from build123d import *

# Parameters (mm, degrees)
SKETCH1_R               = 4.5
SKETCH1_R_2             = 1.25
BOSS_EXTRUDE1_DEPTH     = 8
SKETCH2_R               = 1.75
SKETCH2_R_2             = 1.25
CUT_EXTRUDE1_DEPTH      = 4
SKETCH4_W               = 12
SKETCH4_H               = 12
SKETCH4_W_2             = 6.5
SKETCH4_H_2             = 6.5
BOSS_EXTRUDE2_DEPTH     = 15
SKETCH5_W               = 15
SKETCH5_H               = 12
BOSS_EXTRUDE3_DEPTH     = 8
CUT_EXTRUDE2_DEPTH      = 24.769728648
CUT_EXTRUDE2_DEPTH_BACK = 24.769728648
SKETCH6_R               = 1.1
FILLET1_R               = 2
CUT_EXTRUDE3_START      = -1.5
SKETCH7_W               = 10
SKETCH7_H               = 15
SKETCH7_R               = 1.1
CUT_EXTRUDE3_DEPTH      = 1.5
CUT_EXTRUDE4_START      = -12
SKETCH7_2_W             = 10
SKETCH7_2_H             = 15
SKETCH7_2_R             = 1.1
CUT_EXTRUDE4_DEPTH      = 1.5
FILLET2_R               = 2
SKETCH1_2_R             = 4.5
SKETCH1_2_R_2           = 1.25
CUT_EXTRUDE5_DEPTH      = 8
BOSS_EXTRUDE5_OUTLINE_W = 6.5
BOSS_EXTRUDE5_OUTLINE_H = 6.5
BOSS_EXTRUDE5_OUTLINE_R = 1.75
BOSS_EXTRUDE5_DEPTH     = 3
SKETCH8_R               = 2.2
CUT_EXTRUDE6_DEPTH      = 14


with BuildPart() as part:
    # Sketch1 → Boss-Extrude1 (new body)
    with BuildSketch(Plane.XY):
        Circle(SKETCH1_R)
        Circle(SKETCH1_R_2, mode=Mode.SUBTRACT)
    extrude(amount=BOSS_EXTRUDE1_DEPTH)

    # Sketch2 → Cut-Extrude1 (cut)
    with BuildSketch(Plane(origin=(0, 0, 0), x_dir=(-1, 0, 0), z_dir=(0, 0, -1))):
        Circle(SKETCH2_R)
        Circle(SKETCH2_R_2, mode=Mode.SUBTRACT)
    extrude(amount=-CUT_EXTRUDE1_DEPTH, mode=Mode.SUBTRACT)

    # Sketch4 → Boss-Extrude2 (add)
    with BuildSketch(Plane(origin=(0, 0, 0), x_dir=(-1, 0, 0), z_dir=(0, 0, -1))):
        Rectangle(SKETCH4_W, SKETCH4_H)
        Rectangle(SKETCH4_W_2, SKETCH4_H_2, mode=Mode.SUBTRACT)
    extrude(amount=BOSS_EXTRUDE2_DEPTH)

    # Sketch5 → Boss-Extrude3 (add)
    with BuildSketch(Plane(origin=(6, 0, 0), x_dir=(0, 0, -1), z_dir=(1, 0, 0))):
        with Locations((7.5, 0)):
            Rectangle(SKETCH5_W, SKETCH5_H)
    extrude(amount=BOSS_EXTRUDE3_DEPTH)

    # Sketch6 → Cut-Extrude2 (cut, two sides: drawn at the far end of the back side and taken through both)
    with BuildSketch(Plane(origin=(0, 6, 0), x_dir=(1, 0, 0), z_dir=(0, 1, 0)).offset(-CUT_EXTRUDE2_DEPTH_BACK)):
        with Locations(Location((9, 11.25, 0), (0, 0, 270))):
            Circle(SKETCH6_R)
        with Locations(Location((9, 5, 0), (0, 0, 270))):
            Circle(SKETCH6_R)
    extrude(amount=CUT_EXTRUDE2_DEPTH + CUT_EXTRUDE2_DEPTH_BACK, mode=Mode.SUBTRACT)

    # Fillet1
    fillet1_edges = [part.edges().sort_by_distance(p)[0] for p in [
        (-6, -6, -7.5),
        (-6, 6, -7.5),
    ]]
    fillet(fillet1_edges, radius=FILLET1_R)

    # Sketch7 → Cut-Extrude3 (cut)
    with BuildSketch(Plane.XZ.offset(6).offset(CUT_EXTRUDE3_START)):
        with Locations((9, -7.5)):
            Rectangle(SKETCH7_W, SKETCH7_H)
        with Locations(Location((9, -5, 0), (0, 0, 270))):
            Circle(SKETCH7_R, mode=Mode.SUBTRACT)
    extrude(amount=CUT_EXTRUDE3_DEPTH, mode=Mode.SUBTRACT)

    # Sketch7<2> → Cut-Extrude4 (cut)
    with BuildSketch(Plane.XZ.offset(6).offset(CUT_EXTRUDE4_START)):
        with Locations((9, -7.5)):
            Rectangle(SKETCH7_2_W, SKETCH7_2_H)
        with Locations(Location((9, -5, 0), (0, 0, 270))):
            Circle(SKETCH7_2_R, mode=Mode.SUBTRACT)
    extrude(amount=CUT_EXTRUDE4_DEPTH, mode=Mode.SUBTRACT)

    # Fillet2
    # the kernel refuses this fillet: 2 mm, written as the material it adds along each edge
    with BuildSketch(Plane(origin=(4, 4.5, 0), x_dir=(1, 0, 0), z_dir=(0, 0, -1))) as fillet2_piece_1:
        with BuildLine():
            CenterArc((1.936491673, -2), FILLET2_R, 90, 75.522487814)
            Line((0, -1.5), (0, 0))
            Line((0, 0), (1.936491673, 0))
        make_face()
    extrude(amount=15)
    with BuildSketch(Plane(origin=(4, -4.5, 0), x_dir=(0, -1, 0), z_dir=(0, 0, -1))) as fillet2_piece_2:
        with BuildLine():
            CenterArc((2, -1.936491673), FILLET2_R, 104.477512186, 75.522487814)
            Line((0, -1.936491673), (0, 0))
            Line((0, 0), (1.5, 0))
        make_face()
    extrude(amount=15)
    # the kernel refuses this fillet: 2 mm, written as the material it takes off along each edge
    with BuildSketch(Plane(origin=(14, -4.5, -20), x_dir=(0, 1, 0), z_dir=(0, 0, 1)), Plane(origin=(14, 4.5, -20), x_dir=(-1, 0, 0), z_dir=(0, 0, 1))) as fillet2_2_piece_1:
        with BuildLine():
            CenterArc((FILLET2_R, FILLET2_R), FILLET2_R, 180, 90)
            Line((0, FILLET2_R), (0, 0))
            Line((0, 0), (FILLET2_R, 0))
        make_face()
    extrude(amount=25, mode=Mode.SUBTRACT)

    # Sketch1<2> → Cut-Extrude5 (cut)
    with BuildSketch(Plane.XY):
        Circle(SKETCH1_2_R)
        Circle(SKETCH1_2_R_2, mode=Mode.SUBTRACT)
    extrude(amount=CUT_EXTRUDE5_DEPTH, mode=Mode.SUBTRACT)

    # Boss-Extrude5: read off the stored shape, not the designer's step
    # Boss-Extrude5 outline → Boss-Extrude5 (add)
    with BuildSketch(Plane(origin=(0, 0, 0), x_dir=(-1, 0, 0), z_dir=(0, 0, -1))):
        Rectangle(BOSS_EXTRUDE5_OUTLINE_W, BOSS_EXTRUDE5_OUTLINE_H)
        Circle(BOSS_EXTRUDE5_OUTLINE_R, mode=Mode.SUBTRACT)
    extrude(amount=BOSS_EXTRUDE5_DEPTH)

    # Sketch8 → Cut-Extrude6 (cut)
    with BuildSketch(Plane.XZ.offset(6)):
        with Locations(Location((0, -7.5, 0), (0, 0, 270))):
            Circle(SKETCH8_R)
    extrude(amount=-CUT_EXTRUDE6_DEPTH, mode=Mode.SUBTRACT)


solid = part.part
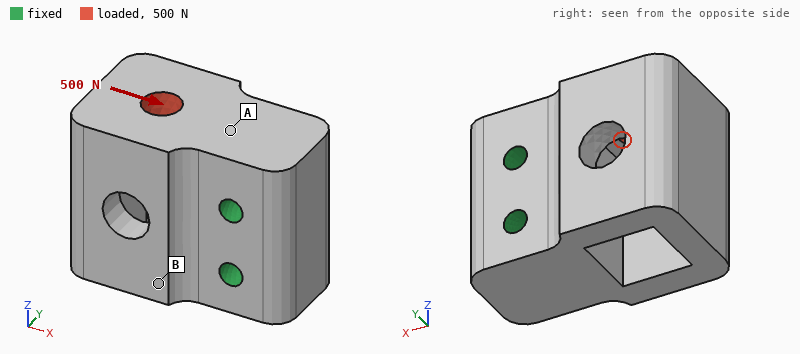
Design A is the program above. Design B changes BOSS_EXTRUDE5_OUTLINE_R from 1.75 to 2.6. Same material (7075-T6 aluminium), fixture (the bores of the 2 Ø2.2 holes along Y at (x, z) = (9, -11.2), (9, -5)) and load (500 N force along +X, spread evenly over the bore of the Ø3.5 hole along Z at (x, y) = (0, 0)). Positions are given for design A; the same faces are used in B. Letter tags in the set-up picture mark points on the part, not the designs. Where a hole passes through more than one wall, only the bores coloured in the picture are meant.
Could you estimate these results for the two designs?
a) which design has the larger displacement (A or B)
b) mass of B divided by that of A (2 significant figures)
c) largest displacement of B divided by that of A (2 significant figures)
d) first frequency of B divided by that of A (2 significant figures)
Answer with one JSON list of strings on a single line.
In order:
["B", "0.99", "1.2", "0.97"]
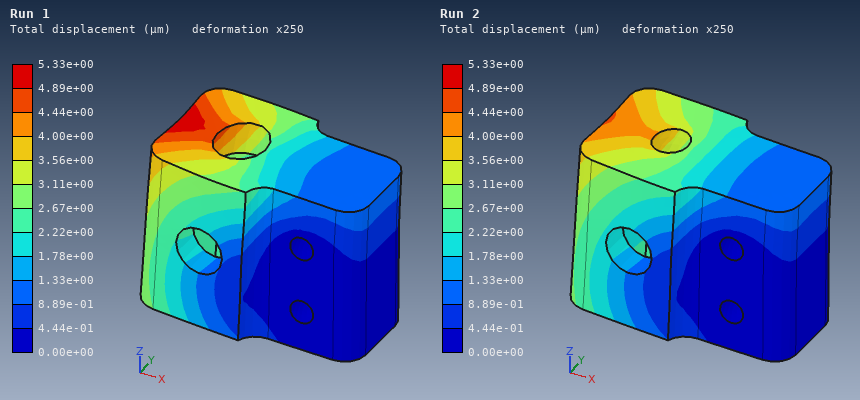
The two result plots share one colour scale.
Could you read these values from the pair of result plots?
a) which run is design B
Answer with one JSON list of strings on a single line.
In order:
["Run 1"]
